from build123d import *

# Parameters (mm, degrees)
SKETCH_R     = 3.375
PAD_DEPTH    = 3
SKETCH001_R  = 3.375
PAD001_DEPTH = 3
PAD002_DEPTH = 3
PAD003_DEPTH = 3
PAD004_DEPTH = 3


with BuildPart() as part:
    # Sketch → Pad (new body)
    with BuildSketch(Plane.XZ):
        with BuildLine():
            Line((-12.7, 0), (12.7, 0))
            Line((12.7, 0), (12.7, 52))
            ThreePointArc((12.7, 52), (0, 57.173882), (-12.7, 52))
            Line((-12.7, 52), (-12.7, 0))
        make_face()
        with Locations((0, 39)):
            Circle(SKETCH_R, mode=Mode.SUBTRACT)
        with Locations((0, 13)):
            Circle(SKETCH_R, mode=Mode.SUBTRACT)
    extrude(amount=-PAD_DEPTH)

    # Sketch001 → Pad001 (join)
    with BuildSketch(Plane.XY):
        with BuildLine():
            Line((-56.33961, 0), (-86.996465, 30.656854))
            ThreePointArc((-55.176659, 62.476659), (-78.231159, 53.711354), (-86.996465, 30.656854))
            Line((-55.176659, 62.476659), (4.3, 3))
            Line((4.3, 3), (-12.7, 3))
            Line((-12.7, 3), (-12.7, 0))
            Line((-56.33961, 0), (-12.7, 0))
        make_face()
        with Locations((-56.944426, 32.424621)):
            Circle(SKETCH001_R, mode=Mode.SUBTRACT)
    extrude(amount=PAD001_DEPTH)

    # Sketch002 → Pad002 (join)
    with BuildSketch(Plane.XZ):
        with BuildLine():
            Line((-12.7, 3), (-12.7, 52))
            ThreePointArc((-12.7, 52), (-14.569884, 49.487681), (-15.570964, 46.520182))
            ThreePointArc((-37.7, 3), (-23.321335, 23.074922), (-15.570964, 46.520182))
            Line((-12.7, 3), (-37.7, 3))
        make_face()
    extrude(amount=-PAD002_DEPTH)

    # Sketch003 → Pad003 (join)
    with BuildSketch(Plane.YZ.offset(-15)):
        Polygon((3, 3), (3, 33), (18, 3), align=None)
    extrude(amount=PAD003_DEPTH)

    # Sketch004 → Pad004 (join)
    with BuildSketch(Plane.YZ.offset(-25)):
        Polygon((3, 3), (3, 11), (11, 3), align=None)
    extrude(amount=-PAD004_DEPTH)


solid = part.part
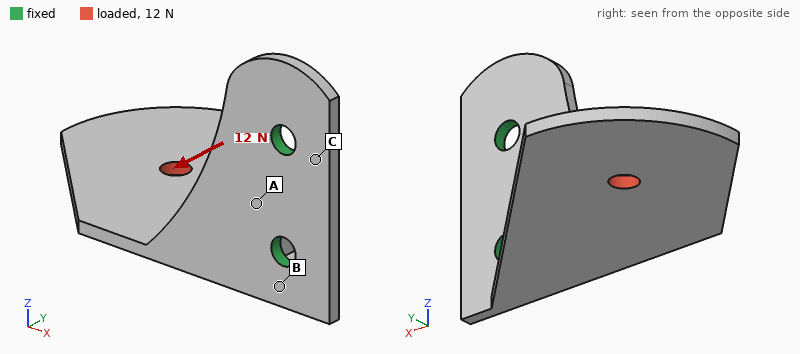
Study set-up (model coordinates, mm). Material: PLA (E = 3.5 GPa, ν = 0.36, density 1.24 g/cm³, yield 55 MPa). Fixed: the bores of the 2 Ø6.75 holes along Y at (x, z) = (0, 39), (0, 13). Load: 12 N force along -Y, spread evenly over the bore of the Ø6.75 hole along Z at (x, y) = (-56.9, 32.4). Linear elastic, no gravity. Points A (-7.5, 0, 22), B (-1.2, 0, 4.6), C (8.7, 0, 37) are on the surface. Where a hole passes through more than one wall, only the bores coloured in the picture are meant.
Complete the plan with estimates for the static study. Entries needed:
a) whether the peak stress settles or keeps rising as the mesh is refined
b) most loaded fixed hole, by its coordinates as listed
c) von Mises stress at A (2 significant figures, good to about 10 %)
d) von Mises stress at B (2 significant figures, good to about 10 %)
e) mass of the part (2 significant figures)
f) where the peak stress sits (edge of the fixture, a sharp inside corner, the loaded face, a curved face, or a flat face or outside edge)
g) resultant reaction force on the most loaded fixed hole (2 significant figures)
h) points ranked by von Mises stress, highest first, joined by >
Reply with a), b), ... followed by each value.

a) keeps rising
b) (0, 13)
c) 5.0 MPa
d) 8.7 MPa
e) 20 g
f) edge of the fixture
g) 20 N
h) B > A > C
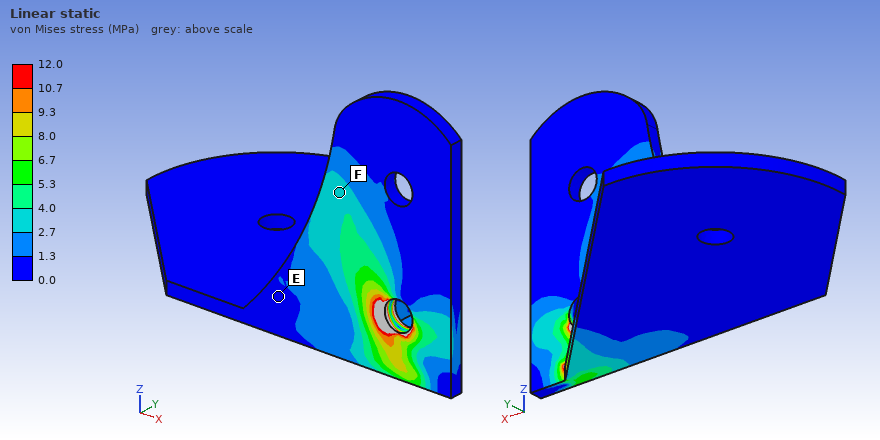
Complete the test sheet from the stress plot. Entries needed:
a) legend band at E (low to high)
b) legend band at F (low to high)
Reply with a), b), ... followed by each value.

a) 0.0 to 1.3 MPa
b) 2.7 to 4.0 MPa
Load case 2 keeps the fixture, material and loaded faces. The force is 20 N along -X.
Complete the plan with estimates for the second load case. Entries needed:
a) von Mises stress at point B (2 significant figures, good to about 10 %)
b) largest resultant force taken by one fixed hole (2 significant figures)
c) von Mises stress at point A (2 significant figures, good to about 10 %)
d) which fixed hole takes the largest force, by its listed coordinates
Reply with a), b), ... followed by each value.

a) 7.7 MPa
b) 24 N
c) 4.5 MPa
d) (0, 13)
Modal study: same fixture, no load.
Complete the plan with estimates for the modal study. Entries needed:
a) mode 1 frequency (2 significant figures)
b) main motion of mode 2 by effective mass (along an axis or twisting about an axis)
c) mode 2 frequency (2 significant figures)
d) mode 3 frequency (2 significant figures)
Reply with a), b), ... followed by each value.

a) 130 Hz
b) along Y
c) 170 Hz
d) 520 Hz
